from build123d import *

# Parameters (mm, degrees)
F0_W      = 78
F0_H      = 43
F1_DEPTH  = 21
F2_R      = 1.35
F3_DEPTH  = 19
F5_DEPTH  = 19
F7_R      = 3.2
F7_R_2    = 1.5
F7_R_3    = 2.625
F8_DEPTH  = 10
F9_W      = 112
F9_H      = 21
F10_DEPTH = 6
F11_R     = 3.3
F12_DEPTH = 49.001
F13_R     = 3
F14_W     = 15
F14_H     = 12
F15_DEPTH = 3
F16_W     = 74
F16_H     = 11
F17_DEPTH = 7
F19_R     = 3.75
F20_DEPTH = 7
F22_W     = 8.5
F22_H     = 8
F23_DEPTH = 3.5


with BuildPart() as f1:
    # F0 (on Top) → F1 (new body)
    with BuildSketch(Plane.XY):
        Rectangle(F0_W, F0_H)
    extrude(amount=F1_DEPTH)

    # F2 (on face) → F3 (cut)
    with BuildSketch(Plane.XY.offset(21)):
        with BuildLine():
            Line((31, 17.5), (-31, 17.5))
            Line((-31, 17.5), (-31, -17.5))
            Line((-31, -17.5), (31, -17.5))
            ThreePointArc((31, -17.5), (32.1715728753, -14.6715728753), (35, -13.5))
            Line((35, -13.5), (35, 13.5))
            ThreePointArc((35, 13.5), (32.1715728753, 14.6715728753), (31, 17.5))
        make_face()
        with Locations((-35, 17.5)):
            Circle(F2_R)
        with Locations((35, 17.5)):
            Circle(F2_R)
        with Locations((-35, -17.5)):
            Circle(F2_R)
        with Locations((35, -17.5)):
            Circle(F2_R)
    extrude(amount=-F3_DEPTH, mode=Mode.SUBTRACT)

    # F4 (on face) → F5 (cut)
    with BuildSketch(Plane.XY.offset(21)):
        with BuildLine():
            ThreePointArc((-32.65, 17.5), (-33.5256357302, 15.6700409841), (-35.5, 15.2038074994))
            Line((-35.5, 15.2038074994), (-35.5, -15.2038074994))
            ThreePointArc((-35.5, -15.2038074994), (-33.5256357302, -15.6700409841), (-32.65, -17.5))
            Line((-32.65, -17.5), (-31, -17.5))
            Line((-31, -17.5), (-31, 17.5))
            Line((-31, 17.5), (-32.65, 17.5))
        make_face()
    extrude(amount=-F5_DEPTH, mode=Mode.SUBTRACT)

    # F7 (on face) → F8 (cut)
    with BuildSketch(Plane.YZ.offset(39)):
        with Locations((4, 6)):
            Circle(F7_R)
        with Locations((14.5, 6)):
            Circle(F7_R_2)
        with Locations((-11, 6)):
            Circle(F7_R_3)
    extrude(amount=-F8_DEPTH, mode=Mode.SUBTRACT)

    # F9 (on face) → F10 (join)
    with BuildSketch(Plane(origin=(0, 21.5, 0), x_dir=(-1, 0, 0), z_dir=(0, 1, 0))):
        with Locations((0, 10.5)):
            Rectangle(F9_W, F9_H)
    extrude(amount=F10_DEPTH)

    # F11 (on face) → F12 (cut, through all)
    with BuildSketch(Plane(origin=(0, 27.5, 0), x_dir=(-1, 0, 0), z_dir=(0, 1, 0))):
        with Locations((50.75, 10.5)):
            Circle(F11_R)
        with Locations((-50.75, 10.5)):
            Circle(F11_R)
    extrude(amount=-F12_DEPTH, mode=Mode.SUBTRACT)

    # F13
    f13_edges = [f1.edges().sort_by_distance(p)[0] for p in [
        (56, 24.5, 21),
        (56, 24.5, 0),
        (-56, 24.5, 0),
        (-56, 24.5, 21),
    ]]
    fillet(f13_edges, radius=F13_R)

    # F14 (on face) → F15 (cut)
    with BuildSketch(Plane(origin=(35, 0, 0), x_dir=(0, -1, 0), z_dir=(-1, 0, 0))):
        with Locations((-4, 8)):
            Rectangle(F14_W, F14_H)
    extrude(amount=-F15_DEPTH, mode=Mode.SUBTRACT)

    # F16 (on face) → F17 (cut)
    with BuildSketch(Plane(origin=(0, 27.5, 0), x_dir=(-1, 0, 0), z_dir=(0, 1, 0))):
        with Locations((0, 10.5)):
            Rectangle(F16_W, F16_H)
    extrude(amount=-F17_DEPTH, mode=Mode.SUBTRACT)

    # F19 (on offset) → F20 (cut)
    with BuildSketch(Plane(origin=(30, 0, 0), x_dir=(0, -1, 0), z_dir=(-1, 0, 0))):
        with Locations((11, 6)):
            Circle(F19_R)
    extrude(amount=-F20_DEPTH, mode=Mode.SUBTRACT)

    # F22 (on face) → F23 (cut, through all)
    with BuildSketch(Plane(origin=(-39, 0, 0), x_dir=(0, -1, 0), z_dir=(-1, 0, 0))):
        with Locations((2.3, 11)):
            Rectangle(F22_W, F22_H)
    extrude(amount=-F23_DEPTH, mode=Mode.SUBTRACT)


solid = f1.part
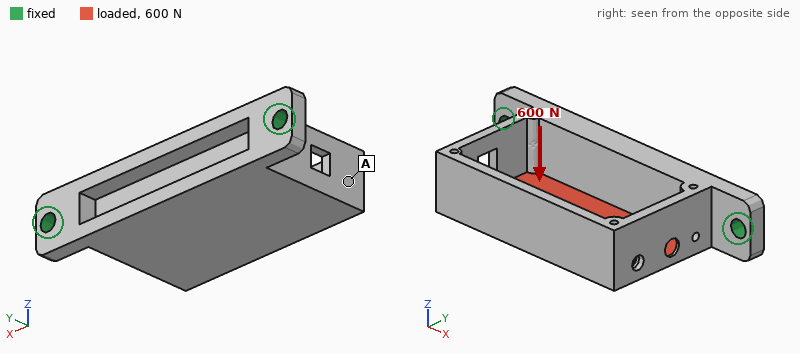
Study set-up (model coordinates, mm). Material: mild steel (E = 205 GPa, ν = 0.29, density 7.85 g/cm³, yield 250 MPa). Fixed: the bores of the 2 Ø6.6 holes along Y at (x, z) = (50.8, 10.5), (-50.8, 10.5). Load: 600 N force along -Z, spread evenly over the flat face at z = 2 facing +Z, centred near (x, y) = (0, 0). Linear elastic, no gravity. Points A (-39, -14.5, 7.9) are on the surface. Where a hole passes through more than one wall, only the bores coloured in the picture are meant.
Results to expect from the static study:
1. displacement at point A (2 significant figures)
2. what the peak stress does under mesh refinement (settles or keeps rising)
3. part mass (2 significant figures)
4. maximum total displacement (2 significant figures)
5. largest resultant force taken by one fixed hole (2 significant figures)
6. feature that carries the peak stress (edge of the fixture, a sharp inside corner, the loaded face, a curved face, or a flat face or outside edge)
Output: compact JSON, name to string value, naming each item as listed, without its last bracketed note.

{"displacement at point A": "35 µm", "what the peak stress does under mesh refinement": "keeps rising", "part mass": "240 g", "maximum total displacement": "43 µm", "largest resultant force taken by one fixed hole": "300 N", "feature that carries the peak stress": "edge of the fixture"}
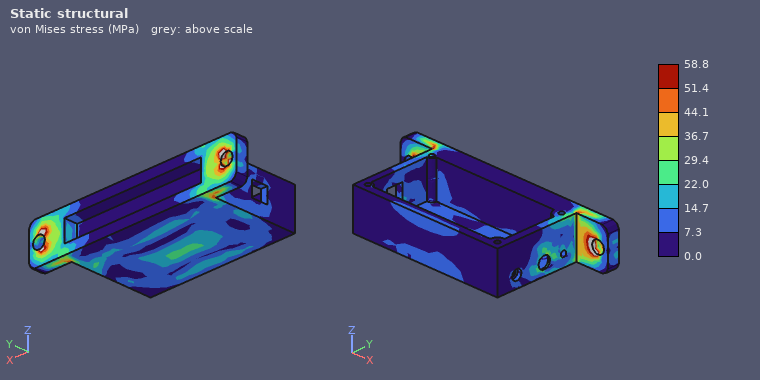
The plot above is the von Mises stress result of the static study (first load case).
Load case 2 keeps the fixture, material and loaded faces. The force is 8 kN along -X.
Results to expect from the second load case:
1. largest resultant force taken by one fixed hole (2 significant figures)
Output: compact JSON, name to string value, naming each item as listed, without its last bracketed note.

{"largest resultant force taken by one fixed hole": "4.7 kN"}
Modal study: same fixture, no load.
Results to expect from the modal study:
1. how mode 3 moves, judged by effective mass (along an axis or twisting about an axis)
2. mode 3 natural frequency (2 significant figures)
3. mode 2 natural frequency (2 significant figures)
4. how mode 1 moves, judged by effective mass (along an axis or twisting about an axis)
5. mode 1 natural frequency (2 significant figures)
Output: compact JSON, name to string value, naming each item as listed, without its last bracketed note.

{"how mode 3 moves, judged by effective mass": "along Y", "mode 3 natural frequency": "4700 Hz", "mode 2 natural frequency": "2600 Hz", "how mode 1 moves, judged by effective mass": "along Z", "mode 1 natural frequency": "1600 Hz"}
